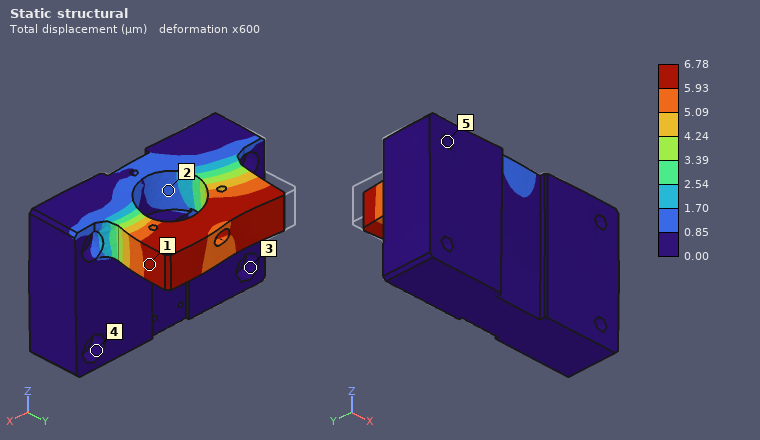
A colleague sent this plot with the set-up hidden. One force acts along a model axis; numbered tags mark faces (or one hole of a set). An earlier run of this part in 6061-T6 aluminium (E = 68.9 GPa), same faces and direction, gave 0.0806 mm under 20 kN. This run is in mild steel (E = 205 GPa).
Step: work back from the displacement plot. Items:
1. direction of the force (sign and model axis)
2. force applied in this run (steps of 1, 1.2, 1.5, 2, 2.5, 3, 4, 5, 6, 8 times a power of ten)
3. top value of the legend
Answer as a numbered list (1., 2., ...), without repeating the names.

1. +X
2. 5 kN
3. 6.78 µm
